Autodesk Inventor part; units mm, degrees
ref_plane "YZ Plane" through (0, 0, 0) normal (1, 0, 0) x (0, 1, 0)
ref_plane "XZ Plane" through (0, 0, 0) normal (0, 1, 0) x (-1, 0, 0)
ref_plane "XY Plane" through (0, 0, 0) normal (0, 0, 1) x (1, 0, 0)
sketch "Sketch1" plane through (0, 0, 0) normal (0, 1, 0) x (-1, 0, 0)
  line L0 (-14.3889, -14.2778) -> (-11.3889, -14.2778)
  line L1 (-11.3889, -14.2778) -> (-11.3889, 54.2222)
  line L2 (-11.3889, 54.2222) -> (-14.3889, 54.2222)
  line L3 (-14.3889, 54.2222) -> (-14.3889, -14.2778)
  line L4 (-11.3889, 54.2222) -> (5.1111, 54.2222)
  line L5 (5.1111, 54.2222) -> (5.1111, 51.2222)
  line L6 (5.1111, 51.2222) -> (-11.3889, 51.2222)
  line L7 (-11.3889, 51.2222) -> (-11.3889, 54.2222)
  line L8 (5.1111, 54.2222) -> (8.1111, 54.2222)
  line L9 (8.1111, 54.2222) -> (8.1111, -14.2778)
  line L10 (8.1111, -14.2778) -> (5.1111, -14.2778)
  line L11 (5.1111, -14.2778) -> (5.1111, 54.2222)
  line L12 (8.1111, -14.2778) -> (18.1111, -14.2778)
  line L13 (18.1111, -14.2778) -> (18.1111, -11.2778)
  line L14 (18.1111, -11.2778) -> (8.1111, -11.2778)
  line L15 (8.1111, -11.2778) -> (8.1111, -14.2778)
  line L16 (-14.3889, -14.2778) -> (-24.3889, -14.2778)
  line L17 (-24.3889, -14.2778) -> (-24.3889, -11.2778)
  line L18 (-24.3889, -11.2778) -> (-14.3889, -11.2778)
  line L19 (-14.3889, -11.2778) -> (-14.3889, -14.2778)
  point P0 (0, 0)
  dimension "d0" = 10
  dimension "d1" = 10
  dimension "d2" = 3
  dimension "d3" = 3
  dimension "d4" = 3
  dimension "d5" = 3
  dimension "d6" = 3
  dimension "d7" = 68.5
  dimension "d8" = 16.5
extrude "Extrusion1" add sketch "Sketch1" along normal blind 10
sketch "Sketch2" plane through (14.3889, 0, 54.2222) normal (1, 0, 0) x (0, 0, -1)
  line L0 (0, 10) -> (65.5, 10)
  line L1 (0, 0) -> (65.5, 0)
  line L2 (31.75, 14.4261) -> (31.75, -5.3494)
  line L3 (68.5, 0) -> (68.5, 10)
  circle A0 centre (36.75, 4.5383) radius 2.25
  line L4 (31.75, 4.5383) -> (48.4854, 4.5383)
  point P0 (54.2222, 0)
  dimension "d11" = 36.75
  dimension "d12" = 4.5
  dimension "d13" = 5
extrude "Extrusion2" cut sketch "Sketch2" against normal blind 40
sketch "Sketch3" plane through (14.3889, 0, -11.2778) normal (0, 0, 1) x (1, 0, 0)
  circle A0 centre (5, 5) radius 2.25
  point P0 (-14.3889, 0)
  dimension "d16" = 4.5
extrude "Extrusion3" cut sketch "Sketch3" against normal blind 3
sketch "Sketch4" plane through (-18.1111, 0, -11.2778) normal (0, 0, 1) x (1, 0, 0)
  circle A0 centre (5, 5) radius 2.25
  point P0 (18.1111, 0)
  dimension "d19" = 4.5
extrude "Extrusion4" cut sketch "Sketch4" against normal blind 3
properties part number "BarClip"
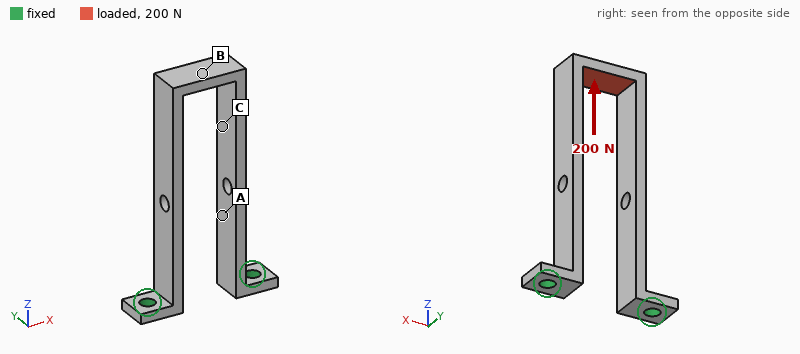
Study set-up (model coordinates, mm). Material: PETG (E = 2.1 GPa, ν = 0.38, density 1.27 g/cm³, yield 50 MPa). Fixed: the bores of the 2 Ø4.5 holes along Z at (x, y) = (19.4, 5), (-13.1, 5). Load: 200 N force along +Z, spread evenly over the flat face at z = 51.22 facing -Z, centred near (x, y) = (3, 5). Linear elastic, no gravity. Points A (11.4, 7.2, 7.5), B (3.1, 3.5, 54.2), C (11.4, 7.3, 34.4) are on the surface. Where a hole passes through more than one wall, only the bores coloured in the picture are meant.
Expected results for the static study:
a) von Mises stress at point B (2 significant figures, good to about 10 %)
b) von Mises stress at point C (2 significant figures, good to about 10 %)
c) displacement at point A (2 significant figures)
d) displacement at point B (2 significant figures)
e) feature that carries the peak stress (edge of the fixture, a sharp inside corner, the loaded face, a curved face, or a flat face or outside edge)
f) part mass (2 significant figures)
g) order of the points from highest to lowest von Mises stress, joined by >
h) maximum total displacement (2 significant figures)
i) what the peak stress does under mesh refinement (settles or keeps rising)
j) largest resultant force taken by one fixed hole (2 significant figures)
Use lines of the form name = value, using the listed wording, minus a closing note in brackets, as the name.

von Mises stress at point B = 25 MPa
von Mises stress at point C = 8.9 MPa
displacement at point A = 0.093 mm
displacement at point B = 0.50 mm
feature that carries the peak stress = edge of the fixture
part mass = 6.4 g
order of the points from highest to lowest von Mises stress, joined by > = B > C > A
maximum total displacement = 0.53 mm
what the peak stress does under mesh refinement = keeps rising
largest resultant force taken by one fixed hole = 100 N
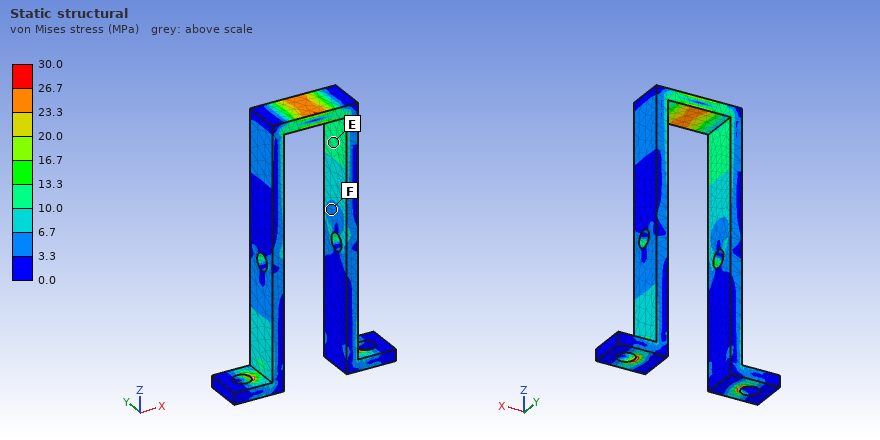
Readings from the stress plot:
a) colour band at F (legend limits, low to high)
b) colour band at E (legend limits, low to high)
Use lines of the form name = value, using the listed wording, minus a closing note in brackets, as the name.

colour band at F = 3.3 to 6.7 MPa
colour band at E = 10.0 to 13.3 MPa
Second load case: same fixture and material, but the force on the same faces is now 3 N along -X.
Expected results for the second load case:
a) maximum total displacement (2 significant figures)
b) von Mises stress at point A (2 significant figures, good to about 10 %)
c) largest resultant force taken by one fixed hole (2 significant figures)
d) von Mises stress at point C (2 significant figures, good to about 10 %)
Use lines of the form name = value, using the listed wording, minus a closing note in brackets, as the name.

maximum total displacement = 0.88 mm
von Mises stress at point A = 1.0 MPa
largest resultant force taken by one fixed hole = 5.1 N
von Mises stress at point C = 1.7 MPa
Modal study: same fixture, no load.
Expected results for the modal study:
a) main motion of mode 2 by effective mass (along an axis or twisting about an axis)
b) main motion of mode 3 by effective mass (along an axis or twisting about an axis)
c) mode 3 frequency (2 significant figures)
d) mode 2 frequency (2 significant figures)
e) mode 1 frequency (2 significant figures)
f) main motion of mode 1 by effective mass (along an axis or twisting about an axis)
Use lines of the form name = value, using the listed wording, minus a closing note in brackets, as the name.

main motion of mode 2 by effective mass = along Y
main motion of mode 3 by effective mass = twisting about Z
mode 3 frequency = 540 Hz
mode 2 frequency = 240 Hz
mode 1 frequency = 180 Hz
main motion of mode 1 by effective mass = along X
